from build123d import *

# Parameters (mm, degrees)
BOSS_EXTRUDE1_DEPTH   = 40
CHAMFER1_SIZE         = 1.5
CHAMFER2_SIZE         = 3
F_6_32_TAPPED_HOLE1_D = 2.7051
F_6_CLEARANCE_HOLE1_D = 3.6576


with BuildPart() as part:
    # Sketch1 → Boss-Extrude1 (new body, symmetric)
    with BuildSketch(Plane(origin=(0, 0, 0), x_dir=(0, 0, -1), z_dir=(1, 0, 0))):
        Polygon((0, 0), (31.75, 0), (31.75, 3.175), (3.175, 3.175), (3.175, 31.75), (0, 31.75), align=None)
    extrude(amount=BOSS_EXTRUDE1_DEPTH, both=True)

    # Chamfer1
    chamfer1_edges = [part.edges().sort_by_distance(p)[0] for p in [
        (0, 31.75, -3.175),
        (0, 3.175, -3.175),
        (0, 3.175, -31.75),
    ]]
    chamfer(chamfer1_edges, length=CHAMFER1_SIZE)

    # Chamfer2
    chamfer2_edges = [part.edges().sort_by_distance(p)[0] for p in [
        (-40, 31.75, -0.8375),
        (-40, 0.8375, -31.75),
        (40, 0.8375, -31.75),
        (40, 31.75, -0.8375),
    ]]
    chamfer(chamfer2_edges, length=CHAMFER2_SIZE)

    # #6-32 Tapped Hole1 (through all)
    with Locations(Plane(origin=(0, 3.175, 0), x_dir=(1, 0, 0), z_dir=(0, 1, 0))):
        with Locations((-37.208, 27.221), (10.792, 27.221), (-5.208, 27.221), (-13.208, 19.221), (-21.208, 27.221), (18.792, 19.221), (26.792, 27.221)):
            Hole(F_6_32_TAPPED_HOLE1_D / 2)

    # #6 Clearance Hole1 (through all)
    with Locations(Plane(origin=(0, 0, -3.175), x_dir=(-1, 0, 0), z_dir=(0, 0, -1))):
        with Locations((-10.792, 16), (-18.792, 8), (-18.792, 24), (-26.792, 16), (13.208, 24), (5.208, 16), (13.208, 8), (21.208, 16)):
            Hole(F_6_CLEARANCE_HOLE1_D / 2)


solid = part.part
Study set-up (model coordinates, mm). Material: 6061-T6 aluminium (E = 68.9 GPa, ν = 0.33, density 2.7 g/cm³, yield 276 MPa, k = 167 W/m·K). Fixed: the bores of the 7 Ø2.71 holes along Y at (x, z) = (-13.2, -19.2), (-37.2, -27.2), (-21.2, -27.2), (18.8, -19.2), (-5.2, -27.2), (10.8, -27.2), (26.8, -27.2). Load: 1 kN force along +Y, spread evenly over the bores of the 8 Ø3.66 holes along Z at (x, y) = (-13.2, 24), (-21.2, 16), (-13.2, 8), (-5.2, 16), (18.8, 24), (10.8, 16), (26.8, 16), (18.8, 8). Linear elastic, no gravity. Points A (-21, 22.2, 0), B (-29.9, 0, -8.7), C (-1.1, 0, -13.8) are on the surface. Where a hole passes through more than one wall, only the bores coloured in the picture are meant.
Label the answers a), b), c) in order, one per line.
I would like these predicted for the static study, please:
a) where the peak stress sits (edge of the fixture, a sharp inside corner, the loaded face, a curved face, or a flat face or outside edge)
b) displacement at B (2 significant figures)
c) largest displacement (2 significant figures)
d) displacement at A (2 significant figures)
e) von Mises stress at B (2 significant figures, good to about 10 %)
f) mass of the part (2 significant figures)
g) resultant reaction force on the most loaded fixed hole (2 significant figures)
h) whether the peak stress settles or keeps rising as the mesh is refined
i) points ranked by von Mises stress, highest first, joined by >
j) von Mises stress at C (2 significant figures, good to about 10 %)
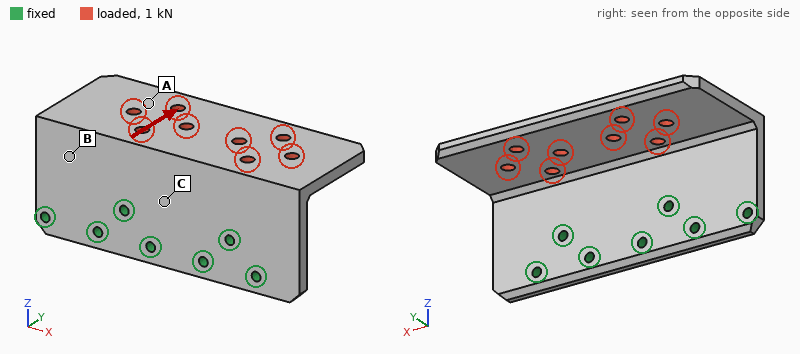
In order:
a) edge of the fixture
b) 0.093 mm
c) 0.44 mm
d) 0.31 mm
e) 42 MPa
f) 40 g
g) 880 N
h) keeps rising
i) C > B > A
j) 77 MPa
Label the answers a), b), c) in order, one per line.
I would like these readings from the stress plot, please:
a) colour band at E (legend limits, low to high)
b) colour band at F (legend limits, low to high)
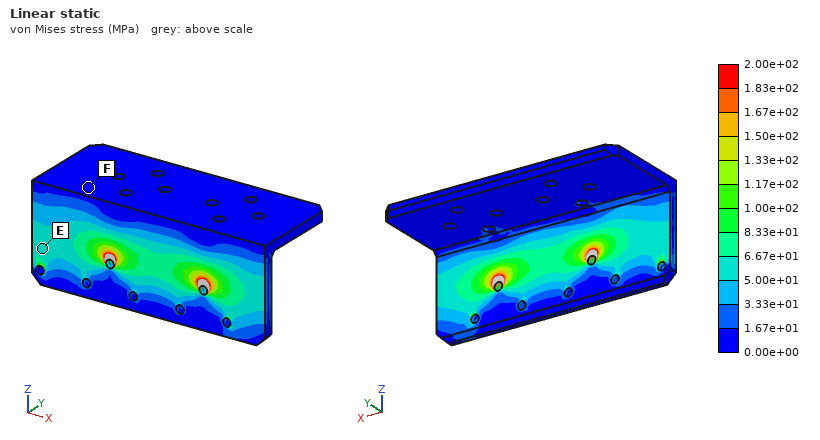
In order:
a) 5.00e+01 to 6.67e+01 MPa
b) 0.00e+00 to 1.67e+01 MPa
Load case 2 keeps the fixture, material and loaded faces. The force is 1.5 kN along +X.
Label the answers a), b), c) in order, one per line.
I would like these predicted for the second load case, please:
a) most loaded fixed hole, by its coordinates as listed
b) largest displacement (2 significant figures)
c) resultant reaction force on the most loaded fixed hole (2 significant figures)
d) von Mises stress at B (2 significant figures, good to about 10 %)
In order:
a) (18.8, -19.2)
b) 0.30 mm
c) 810 N
d) 21 MPa
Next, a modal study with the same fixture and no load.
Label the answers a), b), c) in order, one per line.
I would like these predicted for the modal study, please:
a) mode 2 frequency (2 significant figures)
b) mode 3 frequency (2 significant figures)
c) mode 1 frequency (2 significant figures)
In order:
a) 2100 Hz
b) 3900 Hz
c) 1500 Hz
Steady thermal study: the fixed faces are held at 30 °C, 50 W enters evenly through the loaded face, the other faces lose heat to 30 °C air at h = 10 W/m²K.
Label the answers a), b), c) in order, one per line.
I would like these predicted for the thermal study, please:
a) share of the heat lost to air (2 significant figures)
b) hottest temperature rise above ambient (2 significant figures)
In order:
a) 4.5 %
b) 45 K
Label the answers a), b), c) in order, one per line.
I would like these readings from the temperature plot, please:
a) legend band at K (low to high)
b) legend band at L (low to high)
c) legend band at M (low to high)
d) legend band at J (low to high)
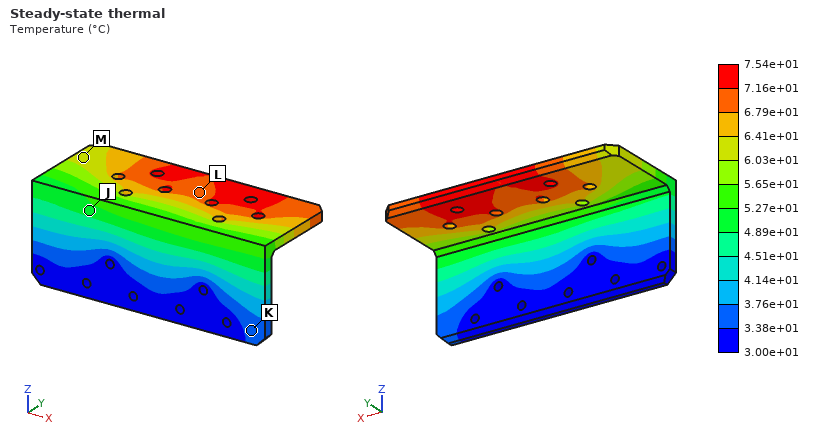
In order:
a) 3.38e+01 to 3.76e+01 °C
b) 6.79e+01 to 7.16e+01 °C
c) 6.03e+01 to 6.41e+01 °C
d) 4.89e+01 to 5.27e+01 °C
